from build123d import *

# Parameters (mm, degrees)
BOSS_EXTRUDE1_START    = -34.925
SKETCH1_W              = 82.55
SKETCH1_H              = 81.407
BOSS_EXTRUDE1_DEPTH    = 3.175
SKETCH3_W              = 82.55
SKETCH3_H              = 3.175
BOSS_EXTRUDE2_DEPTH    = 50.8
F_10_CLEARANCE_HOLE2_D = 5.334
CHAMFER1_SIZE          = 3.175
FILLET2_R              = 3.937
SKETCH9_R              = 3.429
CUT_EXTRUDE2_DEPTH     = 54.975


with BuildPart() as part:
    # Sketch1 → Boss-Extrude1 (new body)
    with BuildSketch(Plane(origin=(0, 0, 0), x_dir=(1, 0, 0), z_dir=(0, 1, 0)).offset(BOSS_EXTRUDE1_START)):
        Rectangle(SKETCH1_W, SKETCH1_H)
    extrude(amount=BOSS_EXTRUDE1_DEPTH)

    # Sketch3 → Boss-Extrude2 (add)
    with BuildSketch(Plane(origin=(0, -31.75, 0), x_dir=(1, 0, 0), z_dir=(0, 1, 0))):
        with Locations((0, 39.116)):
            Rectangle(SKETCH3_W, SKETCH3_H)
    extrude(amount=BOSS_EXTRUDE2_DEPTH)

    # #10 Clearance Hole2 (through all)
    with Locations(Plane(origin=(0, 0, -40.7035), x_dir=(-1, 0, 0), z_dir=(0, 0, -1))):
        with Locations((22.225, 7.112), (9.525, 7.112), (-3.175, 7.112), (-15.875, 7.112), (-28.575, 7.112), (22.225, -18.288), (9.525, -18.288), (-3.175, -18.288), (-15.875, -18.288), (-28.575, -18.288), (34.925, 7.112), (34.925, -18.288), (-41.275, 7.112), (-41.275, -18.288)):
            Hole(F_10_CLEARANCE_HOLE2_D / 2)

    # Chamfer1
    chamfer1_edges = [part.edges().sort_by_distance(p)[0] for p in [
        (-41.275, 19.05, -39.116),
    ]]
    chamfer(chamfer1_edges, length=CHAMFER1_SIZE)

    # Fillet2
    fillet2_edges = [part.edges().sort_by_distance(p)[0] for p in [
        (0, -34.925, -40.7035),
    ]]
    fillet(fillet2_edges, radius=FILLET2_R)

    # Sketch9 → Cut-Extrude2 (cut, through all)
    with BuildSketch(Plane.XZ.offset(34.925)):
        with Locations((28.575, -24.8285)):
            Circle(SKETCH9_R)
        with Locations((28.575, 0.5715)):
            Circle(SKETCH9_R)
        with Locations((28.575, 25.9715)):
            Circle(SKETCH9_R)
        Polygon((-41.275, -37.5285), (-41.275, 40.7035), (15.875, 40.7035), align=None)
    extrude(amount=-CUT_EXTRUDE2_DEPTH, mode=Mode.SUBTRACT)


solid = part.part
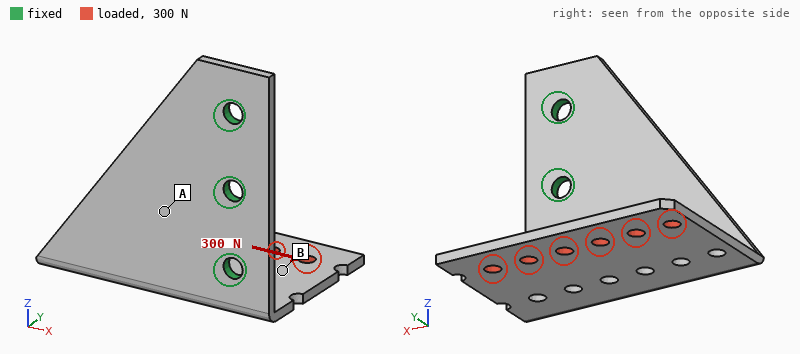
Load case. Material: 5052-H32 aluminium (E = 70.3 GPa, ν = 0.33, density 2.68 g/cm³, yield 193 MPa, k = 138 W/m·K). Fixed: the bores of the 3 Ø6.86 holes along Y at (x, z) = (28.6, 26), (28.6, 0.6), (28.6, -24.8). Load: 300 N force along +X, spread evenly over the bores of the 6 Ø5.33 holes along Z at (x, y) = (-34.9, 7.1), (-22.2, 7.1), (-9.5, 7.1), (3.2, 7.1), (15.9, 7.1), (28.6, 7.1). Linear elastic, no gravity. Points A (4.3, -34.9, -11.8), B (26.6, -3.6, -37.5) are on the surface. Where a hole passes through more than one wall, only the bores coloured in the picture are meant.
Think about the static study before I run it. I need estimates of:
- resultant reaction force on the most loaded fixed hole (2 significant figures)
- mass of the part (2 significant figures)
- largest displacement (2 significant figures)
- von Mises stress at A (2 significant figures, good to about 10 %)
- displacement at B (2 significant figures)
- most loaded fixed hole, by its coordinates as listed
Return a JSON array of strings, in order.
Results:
["360 N", "70 g", "0.95 mm", "34 MPa", "0.32 mm", "(28.6, -24.8)"]
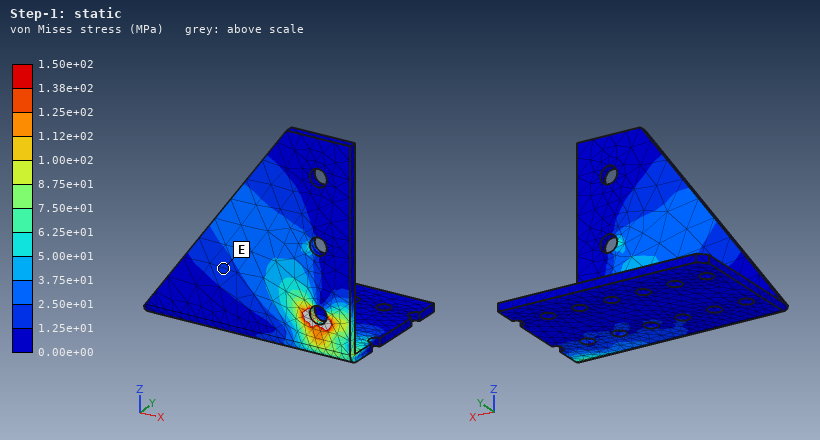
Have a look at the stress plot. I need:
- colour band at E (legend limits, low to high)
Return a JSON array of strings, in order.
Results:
["1.25e+01 to 2.50e+01 MPa"]
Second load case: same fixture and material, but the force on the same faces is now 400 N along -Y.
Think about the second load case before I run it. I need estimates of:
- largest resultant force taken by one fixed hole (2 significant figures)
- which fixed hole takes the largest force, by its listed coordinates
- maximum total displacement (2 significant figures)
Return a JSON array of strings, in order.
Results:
["460 N", "(28.6, -24.8)", "1.1 mm"]
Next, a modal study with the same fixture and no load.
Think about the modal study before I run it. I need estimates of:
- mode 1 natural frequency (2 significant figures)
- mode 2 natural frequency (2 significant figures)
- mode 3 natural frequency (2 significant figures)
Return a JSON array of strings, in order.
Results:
["500 Hz", "680 Hz", "1400 Hz"]
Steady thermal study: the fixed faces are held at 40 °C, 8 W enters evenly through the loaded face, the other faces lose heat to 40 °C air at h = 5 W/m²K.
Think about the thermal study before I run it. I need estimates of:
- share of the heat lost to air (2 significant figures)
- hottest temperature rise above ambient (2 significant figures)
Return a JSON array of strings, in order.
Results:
["9.4 %", "19 K"]
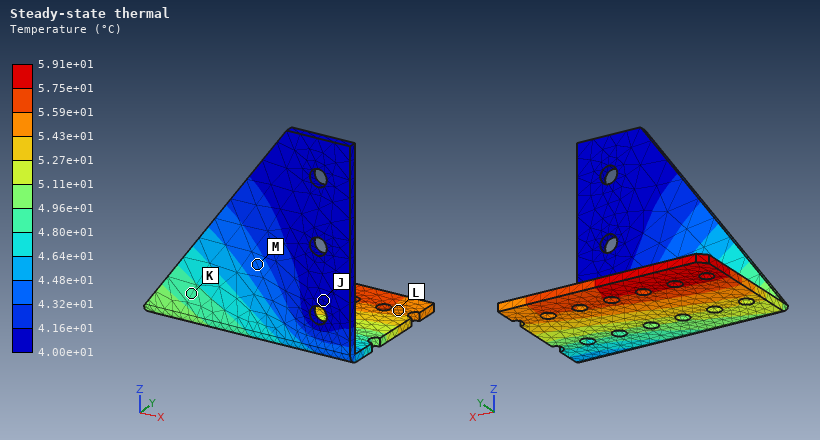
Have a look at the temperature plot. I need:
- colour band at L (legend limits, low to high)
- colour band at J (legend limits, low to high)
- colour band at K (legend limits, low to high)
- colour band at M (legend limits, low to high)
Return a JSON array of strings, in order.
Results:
["5.43e+01 to 5.59e+01 °C", "4.00e+01 to 4.16e+01 °C", "4.80e+01 to 4.96e+01 °C", "4.32e+01 to 4.48e+01 °C"]
